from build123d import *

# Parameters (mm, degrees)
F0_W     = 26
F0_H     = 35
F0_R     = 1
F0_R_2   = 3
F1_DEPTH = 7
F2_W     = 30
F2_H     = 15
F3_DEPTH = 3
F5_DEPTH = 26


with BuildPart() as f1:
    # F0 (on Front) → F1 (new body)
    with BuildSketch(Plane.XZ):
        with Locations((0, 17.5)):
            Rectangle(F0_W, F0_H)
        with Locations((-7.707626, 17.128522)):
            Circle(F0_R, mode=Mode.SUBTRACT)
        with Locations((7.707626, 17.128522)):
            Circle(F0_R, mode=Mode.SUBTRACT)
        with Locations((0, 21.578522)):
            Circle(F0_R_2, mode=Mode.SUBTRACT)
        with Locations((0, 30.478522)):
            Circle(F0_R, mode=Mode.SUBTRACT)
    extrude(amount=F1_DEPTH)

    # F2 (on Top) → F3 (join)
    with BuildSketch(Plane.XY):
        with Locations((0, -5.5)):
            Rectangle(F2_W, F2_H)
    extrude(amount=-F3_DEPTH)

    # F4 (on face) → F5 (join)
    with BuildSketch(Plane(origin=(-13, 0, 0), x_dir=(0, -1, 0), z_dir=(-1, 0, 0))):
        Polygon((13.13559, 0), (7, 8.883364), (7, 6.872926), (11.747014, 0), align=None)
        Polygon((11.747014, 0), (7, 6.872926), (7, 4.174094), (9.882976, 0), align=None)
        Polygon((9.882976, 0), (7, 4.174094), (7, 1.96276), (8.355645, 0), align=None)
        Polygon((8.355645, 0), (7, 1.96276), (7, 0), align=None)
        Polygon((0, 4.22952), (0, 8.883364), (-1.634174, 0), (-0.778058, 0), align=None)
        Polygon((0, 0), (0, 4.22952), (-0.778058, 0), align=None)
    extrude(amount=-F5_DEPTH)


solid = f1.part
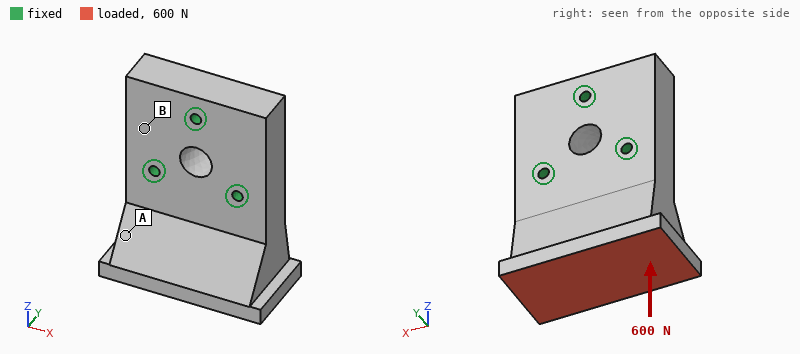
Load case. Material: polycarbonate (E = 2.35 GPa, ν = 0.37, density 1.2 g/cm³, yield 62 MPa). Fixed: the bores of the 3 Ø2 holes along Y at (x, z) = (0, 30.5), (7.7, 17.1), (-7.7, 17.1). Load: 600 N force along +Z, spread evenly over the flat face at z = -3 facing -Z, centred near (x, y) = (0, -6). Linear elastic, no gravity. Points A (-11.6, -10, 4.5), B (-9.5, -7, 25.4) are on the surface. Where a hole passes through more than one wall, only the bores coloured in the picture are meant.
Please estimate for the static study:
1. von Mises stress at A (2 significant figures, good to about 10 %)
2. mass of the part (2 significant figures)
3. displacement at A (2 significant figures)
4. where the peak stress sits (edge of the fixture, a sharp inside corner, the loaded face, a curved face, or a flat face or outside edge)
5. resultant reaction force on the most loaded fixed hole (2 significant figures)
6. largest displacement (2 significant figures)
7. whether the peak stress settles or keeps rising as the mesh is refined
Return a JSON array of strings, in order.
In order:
["3.0 MPa", "10 g", "0.11 mm", "edge of the fixture", "280 N", "0.18 mm", "keeps rising"]
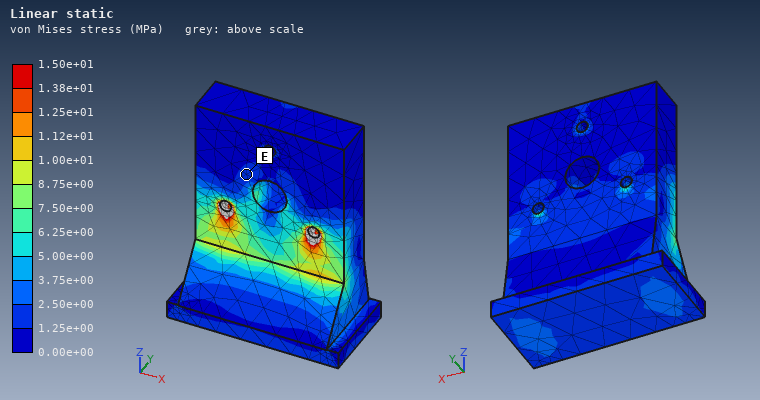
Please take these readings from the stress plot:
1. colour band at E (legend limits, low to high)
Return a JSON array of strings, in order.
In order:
["1.25e+00 to 2.50e+00 MPa"]
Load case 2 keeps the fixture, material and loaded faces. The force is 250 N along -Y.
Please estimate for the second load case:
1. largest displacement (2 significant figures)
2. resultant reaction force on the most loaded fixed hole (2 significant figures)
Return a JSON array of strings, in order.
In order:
["0.55 mm", "170 N"]
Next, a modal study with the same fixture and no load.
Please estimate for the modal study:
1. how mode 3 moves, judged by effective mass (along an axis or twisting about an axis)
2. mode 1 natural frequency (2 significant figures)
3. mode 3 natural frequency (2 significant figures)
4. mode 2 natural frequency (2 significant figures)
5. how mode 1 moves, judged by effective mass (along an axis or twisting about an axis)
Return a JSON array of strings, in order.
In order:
["along X", "2200 Hz", "5200 Hz", "4500 Hz", "along Y"]
